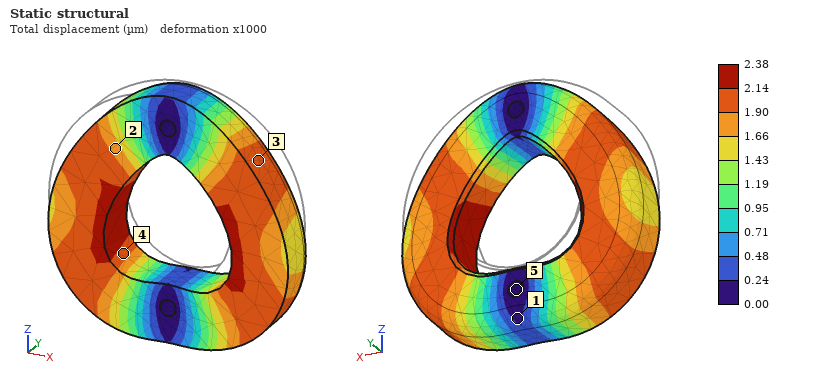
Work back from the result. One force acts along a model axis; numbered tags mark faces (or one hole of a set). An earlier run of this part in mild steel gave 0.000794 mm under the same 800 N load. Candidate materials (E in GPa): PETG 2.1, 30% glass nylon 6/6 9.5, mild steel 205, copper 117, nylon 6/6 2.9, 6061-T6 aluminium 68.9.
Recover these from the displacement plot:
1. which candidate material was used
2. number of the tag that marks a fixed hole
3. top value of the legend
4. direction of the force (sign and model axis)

6061-T6 aluminium
5
2.38 µm
-Z
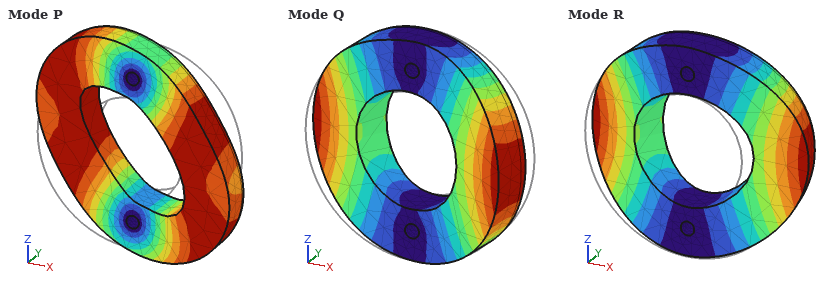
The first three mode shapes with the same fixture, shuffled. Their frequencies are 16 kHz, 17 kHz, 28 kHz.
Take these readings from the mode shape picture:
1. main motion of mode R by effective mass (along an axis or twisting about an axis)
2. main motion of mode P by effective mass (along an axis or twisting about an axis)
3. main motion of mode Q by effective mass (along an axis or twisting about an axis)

along Y
twisting about Y
twisting about Z
